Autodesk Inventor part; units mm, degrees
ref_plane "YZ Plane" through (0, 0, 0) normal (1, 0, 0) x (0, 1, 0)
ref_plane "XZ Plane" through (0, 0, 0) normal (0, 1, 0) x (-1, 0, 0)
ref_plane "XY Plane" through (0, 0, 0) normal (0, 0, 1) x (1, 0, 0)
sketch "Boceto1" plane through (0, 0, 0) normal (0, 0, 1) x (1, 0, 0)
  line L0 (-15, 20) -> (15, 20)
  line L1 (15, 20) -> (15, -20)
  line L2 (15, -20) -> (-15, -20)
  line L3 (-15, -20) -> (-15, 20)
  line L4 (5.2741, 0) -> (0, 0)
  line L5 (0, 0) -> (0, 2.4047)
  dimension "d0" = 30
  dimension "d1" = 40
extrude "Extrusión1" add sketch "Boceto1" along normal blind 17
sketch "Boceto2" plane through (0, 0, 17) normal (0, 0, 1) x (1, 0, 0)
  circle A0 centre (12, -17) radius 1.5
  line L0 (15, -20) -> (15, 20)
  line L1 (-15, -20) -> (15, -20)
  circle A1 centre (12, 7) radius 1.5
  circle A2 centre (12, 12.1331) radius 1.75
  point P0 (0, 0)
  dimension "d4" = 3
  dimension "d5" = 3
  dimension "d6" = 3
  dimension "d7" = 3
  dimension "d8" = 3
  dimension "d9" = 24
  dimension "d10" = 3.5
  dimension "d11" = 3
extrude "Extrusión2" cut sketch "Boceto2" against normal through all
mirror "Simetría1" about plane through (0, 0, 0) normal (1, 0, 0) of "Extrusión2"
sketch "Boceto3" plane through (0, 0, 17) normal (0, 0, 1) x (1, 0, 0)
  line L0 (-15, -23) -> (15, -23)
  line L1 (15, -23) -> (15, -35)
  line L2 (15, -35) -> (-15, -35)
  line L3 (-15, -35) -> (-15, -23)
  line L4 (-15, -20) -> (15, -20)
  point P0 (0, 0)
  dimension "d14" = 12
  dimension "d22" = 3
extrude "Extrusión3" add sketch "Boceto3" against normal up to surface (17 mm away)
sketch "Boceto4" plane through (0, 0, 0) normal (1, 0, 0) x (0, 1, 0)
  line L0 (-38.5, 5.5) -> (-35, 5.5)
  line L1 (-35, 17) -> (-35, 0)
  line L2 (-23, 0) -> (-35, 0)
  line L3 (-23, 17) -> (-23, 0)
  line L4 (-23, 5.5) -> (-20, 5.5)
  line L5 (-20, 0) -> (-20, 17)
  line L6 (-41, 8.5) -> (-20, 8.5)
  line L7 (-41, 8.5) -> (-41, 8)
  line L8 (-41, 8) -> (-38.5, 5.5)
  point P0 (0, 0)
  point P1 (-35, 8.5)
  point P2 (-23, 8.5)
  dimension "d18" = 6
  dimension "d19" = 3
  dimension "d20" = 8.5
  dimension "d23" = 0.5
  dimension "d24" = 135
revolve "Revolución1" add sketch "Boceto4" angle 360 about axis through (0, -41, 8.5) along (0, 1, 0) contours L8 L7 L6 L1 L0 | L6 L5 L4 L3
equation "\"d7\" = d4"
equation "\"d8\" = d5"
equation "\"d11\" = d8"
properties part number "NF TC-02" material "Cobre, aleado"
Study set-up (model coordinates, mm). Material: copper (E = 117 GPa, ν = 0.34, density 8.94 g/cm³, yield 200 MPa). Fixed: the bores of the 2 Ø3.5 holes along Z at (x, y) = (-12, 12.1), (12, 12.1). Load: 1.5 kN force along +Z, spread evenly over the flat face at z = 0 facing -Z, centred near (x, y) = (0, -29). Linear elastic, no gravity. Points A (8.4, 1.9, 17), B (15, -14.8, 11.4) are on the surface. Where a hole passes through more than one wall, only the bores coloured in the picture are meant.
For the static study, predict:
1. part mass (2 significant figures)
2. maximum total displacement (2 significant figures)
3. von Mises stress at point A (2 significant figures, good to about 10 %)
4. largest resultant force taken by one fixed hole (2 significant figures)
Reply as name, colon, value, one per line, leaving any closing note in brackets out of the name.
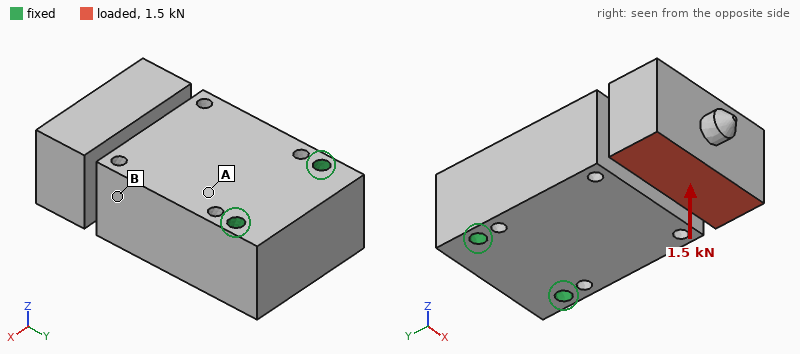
part mass: 230 g
maximum total displacement: 0.22 mm
von Mises stress at point A: 35 MPa
largest resultant force taken by one fixed hole: 750 N
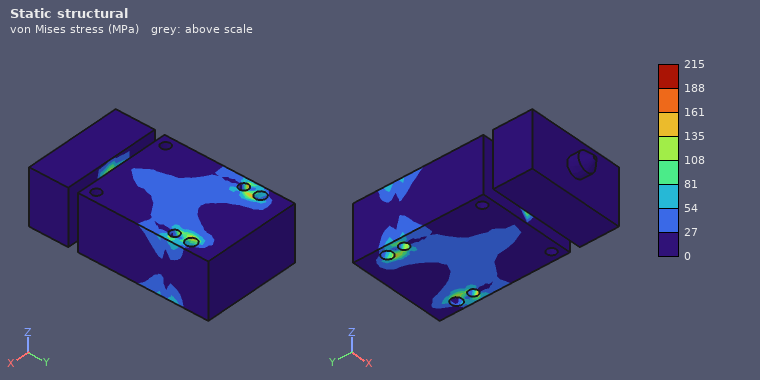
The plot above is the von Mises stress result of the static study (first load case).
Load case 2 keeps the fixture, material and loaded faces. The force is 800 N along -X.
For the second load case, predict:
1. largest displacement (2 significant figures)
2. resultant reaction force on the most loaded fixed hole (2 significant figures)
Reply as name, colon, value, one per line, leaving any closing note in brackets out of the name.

largest displacement: 0.16 mm
resultant reaction force on the most loaded fixed hole: 1.4 kN
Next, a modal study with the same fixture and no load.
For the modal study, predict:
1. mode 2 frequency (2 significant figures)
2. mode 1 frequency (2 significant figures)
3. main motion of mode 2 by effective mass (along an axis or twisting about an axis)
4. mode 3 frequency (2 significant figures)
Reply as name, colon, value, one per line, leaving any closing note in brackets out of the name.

mode 2 frequency: 2200 Hz
mode 1 frequency: 2000 Hz
main motion of mode 2 by effective mass: along Z
mode 3 frequency: 2300 Hz
